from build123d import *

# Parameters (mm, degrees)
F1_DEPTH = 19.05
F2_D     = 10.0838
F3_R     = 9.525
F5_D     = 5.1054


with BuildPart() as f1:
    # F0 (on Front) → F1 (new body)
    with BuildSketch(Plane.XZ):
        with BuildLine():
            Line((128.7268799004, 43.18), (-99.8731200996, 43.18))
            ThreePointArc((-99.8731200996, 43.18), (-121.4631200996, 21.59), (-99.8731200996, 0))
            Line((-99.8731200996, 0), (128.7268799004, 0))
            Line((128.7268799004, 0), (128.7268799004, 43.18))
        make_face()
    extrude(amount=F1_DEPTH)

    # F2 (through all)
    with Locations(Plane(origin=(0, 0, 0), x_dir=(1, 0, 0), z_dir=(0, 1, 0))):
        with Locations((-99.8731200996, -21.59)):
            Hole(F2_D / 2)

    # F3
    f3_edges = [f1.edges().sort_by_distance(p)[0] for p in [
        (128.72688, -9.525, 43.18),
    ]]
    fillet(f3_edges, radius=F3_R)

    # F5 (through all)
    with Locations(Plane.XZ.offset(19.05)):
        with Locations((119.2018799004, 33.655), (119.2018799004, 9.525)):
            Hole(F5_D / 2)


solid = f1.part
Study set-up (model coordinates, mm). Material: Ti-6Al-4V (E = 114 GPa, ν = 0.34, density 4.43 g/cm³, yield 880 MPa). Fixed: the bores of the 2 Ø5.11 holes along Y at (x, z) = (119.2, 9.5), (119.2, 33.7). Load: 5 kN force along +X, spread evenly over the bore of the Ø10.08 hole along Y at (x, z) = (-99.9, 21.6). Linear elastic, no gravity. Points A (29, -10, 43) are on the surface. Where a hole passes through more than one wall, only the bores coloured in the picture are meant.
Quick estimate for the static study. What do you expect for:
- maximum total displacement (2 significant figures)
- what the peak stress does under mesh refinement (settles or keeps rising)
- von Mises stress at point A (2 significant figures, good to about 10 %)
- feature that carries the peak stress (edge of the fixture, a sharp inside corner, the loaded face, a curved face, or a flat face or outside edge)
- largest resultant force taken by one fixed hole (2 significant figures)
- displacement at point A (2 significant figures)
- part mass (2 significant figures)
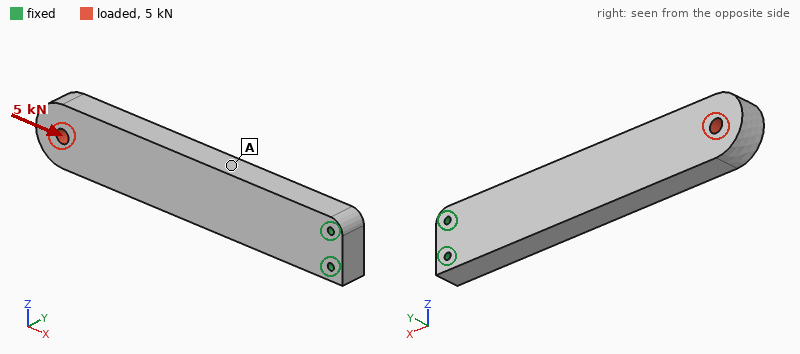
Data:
13 µm
keeps rising
6.1 MPa
edge of the fixture
2.5 kN
5.0 µm
880 g
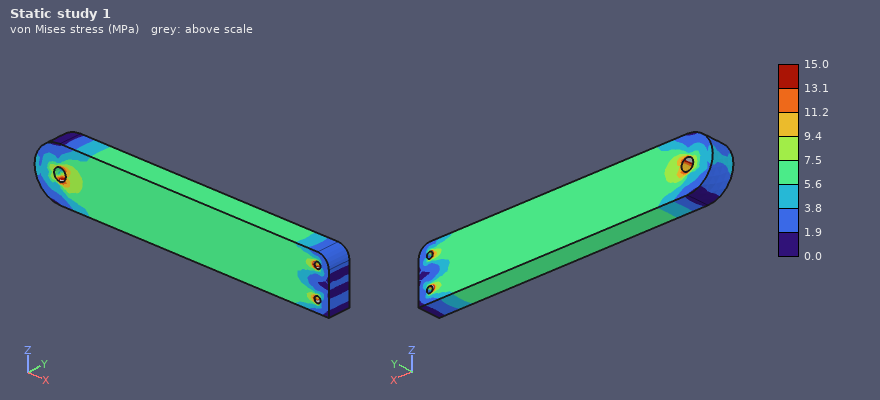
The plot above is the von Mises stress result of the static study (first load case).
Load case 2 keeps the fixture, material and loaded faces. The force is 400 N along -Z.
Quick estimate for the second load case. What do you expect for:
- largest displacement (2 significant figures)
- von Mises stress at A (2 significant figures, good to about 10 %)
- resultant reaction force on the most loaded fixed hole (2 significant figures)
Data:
0.12 mm
8.7 MPa
3.3 kN
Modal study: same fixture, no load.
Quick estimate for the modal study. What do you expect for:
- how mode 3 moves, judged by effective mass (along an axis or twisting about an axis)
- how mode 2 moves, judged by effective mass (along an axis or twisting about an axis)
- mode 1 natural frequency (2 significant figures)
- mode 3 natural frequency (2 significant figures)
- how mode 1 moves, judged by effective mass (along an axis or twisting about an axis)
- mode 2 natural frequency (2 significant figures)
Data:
along Y
along Z
280 Hz
1700 Hz
along Y
610 Hz
